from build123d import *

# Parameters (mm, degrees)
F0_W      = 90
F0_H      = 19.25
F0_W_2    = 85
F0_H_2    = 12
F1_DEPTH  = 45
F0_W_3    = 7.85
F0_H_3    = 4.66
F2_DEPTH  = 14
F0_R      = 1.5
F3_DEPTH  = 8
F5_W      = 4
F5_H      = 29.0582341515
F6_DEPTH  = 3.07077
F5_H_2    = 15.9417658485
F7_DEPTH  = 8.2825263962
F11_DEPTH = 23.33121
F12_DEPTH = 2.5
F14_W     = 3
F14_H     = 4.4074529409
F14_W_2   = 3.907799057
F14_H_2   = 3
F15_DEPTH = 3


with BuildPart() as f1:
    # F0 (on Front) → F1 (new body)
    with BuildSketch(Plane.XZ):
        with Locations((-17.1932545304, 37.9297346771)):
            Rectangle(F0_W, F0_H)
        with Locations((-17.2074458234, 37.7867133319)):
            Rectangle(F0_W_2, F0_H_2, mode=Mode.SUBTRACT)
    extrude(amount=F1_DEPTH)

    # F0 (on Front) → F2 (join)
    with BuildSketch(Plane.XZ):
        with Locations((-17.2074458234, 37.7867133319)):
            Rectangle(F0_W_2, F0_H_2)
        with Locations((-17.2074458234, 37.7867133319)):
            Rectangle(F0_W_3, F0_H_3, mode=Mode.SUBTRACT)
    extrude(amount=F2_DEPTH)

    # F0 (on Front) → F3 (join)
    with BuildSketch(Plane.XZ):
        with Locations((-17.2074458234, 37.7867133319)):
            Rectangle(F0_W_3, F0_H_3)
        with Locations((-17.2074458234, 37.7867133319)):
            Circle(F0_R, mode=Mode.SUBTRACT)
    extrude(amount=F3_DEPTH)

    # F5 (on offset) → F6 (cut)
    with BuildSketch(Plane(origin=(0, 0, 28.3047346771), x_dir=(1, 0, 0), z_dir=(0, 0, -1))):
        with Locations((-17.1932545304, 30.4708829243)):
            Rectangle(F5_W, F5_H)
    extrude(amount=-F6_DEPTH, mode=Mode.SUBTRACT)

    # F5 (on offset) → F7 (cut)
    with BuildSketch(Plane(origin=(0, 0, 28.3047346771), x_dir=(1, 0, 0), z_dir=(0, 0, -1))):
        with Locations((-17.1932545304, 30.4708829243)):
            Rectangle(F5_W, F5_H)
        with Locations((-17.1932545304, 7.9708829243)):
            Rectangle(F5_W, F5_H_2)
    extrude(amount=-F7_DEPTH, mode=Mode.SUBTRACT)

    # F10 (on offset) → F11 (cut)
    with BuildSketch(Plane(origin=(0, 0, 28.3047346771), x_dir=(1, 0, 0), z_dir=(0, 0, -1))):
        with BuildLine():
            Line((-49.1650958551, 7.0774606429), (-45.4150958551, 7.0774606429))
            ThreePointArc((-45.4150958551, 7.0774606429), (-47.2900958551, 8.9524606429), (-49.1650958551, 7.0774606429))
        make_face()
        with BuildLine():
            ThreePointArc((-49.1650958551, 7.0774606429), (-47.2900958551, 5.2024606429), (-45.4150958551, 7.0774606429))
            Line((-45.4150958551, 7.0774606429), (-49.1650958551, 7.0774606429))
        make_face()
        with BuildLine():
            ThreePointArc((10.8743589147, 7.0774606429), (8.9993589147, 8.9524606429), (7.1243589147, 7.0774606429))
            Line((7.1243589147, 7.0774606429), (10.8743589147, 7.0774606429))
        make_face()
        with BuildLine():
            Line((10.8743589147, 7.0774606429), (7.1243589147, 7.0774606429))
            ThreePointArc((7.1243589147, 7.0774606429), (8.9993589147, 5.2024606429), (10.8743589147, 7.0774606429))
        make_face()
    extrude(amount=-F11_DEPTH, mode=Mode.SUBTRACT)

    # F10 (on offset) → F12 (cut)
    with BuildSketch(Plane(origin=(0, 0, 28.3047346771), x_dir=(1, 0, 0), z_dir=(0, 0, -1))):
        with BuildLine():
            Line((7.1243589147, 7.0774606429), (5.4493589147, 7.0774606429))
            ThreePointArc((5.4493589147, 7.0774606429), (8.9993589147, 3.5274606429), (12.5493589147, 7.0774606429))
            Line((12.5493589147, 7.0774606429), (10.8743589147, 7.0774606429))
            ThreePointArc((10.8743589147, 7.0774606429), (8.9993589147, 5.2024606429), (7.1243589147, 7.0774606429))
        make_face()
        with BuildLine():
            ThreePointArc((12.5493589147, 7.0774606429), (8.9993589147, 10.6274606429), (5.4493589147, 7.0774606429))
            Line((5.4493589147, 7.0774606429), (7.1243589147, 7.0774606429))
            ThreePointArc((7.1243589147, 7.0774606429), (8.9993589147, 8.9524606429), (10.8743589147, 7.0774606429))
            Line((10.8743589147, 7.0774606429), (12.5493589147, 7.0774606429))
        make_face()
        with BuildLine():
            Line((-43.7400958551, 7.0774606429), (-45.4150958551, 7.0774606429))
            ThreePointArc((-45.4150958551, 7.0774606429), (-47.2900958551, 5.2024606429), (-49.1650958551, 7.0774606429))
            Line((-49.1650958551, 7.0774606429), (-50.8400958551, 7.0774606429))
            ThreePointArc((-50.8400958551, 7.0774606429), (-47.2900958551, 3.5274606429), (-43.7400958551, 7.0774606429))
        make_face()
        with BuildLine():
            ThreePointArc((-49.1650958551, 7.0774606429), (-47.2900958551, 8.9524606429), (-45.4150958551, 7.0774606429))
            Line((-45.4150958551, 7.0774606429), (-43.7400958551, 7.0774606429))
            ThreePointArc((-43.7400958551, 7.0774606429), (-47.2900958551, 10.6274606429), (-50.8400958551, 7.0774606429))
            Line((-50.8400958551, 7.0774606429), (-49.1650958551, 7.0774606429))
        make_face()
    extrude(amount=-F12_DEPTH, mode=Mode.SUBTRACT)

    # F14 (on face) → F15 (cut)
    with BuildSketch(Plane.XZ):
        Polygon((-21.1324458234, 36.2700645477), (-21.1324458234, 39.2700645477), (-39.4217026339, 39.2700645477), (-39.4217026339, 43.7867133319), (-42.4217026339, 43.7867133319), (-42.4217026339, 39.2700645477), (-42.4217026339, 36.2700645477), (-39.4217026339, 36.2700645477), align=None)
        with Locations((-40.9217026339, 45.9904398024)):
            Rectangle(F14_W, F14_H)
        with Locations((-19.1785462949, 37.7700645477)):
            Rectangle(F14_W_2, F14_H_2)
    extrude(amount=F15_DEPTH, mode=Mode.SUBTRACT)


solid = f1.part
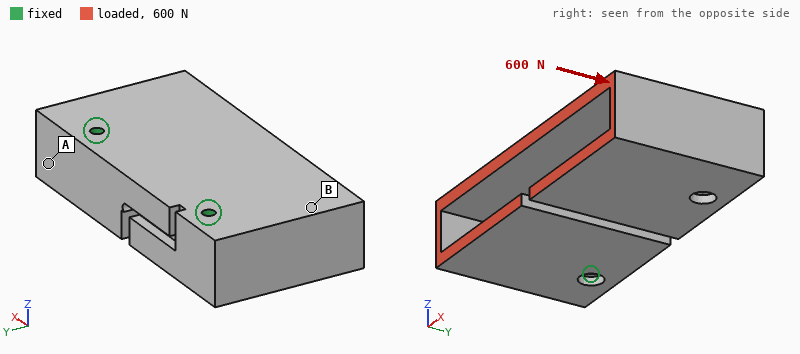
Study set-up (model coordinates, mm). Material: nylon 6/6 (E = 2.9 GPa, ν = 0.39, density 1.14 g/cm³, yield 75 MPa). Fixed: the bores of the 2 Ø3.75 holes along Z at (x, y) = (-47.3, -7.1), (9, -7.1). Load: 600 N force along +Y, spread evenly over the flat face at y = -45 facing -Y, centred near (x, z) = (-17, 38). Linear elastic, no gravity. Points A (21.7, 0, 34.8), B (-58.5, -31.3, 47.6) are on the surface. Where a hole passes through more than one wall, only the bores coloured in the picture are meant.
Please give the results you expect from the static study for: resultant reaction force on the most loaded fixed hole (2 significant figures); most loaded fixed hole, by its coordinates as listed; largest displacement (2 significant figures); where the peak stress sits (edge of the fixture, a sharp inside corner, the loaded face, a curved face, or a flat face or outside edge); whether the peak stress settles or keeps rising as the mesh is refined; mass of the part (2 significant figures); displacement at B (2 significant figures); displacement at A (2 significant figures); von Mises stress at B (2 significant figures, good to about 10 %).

320 N
(9, -7.1)
37 µm
edge of the fixture
keeps rising
51 g
11 µm
8.4 µm
0.94 MPa
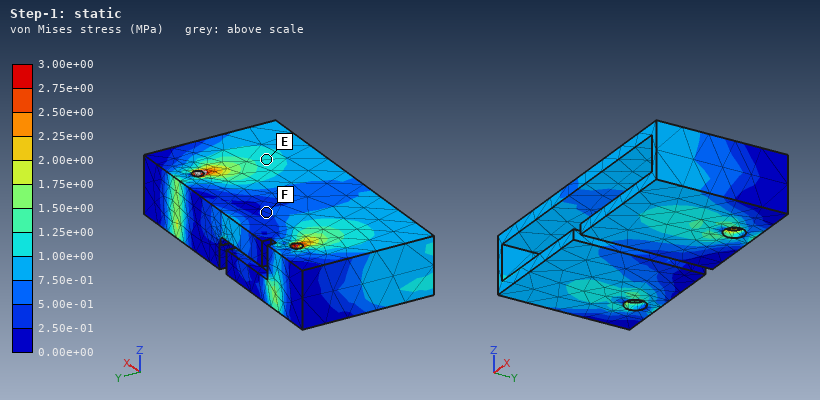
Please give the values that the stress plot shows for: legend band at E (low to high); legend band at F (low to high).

1.00e+00 to 1.25e+00 MPa
2.50e-01 to 5.00e-01 MPa
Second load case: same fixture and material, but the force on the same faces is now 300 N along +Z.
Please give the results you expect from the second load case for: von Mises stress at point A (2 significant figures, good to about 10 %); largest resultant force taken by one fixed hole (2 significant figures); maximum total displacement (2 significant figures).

2.7 MPa
170 N
1.1 mm
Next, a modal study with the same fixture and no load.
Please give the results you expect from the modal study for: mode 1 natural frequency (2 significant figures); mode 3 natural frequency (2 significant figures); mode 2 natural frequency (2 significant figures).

1100 Hz
1300 Hz
1200 Hz
